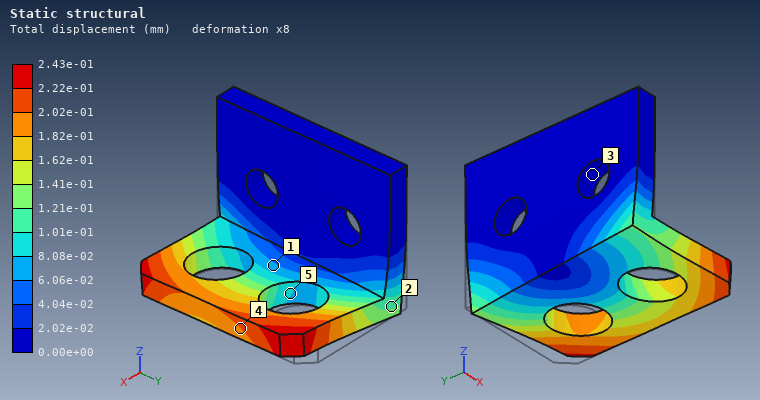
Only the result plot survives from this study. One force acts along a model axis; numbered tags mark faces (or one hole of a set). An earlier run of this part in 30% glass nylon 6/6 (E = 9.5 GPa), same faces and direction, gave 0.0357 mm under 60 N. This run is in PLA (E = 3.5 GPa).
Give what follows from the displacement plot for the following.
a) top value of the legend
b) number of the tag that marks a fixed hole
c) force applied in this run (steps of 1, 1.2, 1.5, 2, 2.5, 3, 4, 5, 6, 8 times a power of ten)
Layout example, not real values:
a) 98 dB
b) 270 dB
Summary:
a) 2.43e-01 mm
b) 3
c) 150 N
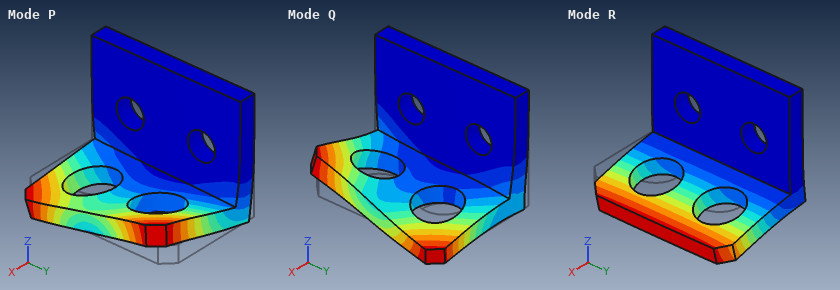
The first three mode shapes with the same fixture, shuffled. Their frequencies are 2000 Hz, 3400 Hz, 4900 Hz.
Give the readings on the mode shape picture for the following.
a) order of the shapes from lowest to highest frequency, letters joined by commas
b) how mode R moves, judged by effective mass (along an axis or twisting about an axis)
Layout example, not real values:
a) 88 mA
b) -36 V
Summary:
a) R, P, Q
b) along Z
